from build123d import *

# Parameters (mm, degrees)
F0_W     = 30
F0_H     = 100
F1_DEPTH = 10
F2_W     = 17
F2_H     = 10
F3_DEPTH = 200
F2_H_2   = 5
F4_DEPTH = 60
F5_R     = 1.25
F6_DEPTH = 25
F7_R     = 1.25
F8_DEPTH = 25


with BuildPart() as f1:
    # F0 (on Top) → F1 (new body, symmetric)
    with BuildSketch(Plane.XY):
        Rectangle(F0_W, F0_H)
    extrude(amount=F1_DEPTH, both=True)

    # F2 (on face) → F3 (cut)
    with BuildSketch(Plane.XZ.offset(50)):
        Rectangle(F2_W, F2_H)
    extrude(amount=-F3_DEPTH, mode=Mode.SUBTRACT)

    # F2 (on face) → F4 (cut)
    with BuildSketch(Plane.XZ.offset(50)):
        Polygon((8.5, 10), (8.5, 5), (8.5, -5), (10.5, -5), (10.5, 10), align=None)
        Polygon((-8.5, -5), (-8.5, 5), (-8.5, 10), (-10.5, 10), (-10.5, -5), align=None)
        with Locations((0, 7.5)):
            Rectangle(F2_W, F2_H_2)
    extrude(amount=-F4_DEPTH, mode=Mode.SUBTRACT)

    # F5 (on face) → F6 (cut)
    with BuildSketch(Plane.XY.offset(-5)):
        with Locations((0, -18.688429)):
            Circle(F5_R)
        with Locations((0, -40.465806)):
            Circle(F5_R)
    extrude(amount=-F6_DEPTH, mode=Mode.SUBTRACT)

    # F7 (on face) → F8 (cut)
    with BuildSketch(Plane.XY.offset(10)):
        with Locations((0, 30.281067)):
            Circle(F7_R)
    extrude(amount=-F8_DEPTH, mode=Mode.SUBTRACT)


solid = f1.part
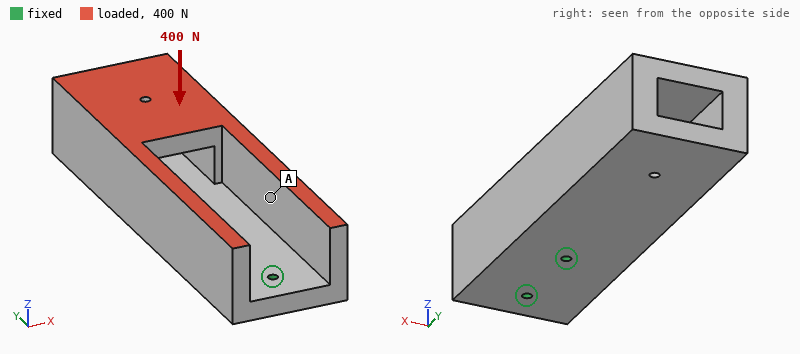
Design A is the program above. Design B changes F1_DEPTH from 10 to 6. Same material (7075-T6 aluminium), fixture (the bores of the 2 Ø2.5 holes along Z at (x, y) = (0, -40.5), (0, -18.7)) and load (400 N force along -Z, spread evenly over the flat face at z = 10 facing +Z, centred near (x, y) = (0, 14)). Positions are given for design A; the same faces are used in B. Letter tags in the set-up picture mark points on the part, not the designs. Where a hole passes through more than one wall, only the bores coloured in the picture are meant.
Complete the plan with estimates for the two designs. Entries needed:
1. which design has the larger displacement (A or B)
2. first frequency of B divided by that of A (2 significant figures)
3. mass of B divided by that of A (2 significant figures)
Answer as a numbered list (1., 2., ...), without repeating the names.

1. B
2. 0.30
3. 0.45
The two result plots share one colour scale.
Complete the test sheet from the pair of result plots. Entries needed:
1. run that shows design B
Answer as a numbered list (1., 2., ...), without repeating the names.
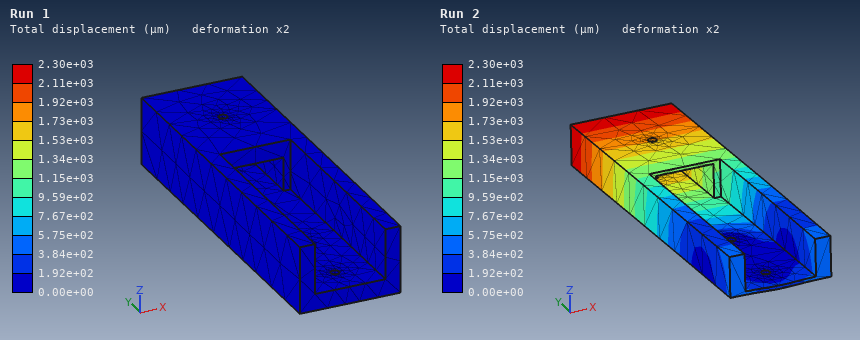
1. Run 2
